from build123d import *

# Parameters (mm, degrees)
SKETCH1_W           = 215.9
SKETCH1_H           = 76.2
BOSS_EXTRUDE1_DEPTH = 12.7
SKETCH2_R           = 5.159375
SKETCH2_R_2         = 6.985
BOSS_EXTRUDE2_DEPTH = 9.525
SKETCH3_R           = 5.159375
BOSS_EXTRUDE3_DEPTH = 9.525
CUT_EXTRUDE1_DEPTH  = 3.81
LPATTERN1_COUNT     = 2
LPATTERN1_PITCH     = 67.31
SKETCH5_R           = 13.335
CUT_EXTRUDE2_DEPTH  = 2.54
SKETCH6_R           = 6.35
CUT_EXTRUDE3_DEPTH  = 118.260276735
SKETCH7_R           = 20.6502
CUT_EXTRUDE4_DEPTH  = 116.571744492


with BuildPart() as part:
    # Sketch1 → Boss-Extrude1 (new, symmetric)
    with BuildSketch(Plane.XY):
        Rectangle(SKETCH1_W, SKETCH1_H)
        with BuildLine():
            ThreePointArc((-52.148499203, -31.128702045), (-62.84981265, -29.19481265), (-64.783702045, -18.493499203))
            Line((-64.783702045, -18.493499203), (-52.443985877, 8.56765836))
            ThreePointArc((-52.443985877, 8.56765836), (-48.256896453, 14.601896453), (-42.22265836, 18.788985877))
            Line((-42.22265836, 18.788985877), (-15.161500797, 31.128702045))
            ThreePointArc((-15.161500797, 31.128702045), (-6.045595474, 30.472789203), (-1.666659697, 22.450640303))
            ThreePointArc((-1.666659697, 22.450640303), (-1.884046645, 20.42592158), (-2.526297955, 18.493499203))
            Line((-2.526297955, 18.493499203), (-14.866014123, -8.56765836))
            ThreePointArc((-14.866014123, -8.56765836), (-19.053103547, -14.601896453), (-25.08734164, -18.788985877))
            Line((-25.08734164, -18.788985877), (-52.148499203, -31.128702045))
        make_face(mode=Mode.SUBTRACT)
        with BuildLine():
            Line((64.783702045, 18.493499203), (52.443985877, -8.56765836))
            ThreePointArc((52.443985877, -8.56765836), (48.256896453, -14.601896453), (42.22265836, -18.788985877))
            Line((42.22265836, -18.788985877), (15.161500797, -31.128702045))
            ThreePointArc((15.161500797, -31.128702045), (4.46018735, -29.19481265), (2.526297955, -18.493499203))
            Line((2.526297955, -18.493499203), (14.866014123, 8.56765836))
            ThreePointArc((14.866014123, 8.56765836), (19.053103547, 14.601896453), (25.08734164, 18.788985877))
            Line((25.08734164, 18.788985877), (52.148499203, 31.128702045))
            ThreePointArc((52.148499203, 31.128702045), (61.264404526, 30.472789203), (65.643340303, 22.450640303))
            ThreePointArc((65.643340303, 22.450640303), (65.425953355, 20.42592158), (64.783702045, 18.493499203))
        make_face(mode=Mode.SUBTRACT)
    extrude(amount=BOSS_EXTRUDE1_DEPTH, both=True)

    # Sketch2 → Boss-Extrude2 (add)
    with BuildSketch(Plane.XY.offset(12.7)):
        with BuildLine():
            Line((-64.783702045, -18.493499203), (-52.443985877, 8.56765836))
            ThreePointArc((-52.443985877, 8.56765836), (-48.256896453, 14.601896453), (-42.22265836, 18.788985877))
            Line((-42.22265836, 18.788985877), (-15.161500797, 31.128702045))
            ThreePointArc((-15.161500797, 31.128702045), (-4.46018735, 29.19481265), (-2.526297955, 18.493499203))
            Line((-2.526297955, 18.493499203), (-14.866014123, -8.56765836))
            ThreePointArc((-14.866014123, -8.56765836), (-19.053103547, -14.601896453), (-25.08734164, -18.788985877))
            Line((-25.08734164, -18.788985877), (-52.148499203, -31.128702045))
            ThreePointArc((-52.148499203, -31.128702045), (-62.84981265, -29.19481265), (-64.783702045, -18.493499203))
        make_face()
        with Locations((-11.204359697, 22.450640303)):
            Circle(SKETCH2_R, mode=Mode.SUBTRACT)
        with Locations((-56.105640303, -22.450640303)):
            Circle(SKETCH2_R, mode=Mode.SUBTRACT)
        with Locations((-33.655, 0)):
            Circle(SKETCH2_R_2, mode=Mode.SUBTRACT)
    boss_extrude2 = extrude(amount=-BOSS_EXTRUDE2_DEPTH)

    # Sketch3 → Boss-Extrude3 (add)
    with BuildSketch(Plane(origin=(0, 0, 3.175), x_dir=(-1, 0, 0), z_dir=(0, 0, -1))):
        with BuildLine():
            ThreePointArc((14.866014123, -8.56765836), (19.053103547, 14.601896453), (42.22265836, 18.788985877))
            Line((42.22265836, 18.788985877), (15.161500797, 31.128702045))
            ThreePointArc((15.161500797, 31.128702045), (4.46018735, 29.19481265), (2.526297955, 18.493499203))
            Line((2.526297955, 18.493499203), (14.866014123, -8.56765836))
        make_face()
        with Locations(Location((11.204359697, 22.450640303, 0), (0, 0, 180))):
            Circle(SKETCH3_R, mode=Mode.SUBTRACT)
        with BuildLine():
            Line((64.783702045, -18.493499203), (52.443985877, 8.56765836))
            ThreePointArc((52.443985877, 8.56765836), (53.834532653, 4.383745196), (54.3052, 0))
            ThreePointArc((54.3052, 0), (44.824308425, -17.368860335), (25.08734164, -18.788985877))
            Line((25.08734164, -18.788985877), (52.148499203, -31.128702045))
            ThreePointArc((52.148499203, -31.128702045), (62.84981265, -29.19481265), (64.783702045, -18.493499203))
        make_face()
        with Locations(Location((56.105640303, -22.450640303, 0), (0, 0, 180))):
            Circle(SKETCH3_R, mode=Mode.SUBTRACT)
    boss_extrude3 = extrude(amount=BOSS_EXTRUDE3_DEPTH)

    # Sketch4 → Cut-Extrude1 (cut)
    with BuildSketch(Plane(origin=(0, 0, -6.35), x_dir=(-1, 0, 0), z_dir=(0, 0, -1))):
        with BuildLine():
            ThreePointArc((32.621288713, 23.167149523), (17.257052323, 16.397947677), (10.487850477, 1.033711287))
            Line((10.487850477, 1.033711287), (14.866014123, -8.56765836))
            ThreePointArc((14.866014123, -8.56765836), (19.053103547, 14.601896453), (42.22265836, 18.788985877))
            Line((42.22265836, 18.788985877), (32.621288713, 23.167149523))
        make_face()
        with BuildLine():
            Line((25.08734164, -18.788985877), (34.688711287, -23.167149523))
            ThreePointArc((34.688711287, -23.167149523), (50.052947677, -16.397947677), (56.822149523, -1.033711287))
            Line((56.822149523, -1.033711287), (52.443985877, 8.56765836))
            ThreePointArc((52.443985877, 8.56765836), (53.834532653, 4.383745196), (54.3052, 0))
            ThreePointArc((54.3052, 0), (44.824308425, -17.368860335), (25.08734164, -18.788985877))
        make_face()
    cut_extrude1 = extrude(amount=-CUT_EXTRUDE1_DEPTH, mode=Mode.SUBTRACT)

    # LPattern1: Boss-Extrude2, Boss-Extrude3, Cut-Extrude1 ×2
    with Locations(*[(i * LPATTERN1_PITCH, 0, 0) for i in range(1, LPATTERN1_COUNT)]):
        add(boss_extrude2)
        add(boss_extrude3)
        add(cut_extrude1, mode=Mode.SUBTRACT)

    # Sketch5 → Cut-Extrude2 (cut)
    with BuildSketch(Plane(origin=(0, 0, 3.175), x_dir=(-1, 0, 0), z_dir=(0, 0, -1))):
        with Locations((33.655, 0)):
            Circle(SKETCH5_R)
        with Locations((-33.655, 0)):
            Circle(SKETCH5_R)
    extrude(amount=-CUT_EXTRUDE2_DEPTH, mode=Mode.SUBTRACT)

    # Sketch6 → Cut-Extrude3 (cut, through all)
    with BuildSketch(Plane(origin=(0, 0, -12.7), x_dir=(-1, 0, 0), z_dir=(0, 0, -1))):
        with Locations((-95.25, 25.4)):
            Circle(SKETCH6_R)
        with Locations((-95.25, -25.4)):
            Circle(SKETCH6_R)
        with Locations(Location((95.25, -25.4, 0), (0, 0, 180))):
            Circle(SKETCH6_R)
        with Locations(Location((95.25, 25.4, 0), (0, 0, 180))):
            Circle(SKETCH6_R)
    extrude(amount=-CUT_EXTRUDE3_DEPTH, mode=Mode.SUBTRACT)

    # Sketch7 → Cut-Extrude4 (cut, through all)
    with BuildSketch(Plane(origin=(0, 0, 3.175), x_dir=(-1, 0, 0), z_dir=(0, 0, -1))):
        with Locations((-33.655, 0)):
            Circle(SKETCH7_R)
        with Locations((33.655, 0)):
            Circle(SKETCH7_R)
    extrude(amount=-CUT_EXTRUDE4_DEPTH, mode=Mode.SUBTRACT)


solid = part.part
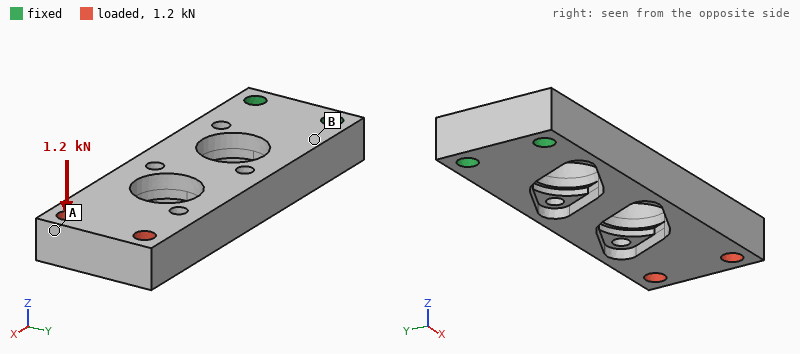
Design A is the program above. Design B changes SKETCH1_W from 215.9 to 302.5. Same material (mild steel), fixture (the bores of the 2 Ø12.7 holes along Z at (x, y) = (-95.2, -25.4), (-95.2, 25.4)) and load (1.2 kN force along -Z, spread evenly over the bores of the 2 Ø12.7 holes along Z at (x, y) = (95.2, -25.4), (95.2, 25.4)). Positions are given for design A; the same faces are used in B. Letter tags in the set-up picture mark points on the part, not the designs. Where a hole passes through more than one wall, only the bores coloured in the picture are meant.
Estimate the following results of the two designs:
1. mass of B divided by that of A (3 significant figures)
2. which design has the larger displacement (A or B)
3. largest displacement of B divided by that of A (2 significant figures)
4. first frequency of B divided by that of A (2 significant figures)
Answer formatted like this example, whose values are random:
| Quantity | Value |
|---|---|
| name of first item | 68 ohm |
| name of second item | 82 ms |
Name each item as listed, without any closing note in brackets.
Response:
| Quantity | Value |
|---|---|
| mass of B divided by that of A | 1.53 |
| which design has the larger displacement | B |
| largest displacement of B divided by that of A | 1.3 |
| first frequency of B divided by that of A | 0.63 |
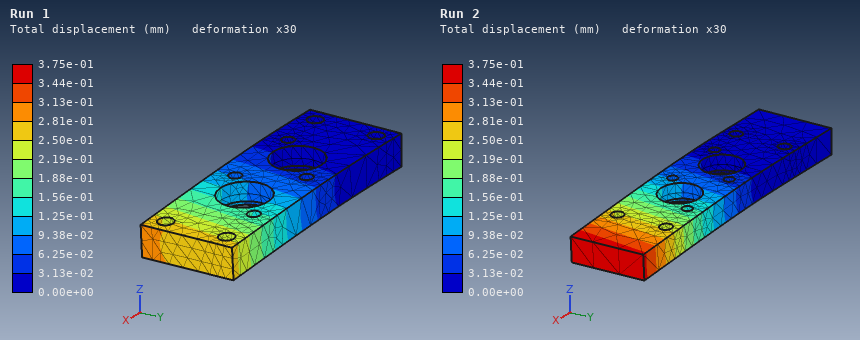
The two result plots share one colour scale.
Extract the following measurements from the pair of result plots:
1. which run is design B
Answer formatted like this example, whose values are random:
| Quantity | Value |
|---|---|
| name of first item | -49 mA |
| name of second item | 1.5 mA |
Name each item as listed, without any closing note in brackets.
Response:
| Quantity | Value |
|---|---|
| which run is design B | Run 2 |
